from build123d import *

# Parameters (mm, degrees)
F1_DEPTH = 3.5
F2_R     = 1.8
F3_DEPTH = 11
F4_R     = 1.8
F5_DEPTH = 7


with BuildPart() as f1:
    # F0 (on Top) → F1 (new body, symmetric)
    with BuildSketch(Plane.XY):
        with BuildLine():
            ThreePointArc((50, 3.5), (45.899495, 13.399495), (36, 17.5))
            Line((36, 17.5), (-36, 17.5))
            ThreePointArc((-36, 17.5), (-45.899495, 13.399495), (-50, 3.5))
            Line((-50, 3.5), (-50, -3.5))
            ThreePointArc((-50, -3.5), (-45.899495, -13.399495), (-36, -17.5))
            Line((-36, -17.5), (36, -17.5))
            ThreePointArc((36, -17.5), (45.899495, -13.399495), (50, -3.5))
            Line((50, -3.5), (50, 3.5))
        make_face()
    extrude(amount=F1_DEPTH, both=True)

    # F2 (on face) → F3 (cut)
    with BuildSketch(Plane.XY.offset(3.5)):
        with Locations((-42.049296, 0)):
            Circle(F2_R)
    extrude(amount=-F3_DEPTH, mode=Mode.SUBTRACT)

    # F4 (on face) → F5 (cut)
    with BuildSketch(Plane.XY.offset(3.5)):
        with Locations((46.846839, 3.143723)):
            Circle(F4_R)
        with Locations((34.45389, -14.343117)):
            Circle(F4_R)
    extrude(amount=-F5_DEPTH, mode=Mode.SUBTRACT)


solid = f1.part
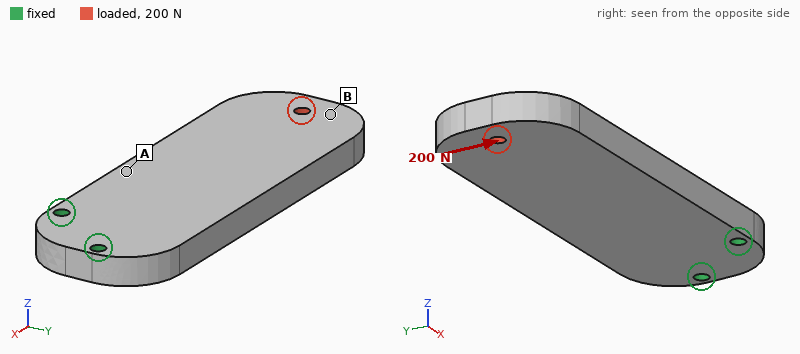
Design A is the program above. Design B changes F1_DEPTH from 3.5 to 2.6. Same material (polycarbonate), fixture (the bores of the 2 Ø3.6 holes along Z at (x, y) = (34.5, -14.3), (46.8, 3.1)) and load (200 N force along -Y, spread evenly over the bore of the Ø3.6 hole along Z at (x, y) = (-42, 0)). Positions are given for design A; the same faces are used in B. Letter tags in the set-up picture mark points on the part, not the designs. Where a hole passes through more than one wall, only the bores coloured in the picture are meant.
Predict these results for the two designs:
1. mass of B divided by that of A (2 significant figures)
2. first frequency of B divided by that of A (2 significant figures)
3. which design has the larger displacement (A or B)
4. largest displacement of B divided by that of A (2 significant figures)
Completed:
0.74
0.75
B
1.3
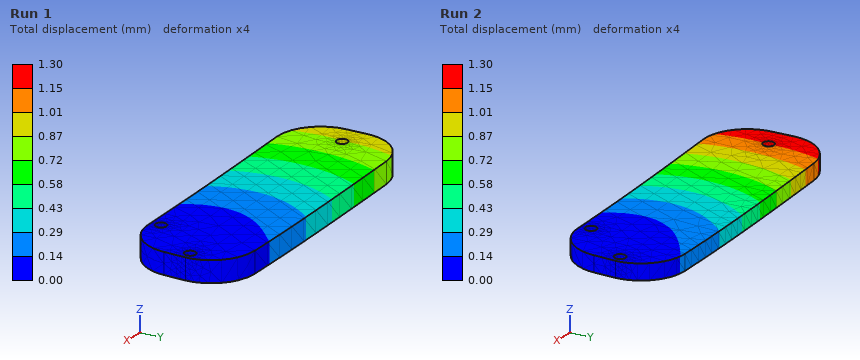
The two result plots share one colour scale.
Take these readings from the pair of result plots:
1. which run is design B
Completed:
Run 2
